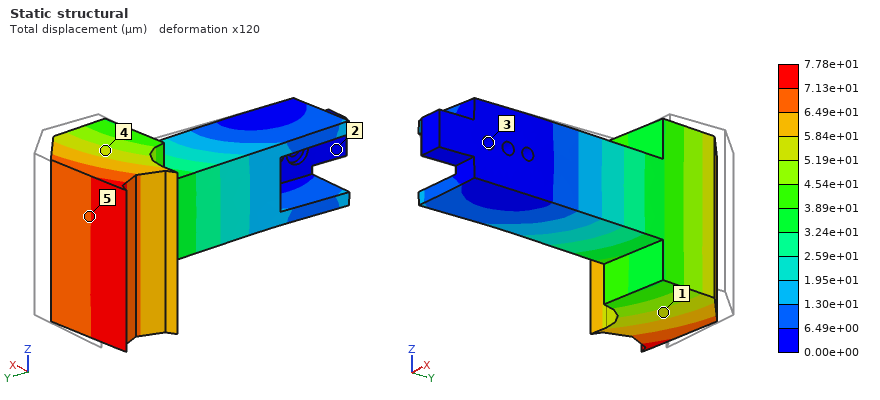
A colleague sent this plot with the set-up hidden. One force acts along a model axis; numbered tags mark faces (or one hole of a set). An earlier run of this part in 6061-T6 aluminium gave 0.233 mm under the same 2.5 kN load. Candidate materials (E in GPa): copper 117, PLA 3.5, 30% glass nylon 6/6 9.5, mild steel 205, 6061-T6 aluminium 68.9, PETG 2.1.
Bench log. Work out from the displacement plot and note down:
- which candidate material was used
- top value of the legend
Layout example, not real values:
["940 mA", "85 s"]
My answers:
["mild steel", "7.78e+01 µm"]
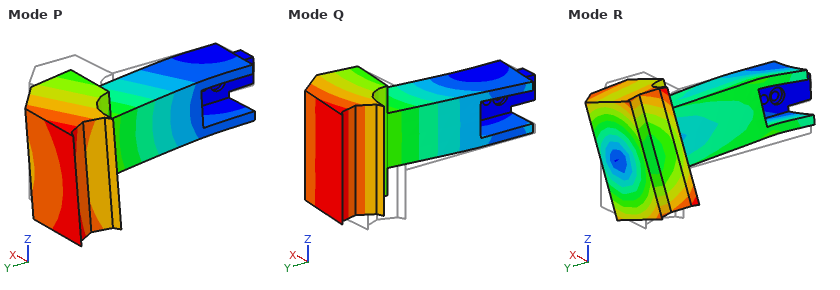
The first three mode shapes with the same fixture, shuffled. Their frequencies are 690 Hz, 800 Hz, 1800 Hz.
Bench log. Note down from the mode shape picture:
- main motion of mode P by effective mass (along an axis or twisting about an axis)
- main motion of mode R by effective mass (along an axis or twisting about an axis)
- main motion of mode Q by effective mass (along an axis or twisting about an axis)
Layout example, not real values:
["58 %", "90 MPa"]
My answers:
["along Z", "twisting about Y", "along X"]
